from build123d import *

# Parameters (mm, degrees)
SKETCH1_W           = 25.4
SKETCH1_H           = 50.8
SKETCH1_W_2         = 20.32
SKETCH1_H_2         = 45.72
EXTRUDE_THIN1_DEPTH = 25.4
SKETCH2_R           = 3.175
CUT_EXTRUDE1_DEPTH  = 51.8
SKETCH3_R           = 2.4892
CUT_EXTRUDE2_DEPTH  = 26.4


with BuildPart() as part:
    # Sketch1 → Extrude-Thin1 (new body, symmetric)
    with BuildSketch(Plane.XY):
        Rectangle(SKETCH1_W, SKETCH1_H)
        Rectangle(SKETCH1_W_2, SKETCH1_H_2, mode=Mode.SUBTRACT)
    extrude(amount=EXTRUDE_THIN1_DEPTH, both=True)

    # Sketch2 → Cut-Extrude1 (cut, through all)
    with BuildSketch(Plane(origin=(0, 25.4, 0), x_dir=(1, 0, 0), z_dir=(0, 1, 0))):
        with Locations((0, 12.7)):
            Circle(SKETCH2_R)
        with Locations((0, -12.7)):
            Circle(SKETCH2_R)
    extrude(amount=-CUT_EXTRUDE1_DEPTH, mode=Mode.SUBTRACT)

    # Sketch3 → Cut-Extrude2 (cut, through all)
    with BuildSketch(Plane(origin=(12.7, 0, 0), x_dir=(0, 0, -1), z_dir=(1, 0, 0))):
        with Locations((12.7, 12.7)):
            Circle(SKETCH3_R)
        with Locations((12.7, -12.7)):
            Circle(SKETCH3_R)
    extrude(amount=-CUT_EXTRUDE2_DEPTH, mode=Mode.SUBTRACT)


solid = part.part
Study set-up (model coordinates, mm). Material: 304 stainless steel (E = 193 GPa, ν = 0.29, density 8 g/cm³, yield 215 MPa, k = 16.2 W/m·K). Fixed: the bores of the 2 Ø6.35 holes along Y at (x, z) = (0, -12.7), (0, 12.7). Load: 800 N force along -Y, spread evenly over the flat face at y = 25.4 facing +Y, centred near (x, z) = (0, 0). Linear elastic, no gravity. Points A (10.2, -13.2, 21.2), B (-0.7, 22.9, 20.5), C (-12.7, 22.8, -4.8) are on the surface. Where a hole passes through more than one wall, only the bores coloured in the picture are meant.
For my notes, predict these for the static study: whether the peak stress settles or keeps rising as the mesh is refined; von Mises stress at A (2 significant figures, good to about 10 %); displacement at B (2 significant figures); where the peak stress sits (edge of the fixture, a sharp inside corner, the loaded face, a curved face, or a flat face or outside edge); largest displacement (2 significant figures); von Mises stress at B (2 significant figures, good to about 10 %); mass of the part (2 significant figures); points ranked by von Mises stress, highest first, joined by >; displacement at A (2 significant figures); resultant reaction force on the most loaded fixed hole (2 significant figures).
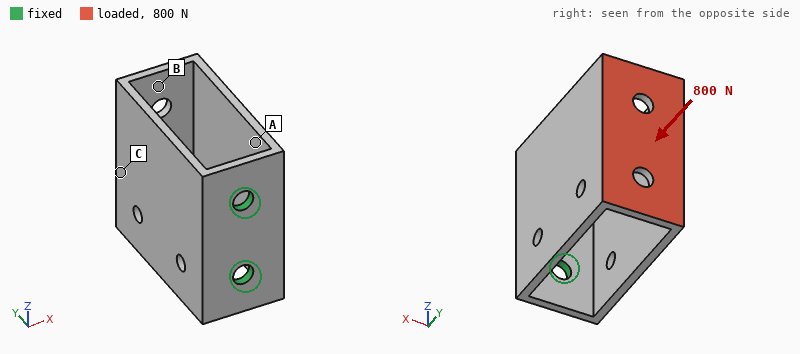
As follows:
keeps rising
13 MPa
15 µm
edge of the fixture
16 µm
33 MPa
140 g
B > A > C
11 µm
400 N
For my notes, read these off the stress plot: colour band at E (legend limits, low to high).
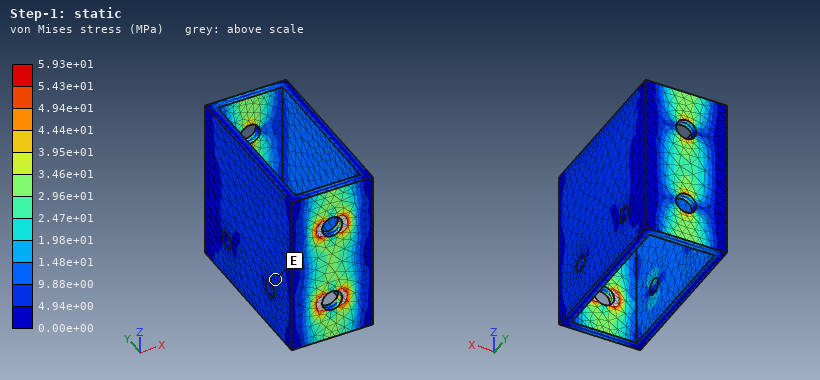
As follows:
4.94e+00 to 9.88e+00 MPa
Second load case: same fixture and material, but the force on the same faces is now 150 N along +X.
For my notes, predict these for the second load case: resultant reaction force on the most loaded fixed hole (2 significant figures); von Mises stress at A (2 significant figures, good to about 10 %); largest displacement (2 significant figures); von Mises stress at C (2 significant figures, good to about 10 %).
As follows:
75 N
15 MPa
0.13 mm
24 MPa
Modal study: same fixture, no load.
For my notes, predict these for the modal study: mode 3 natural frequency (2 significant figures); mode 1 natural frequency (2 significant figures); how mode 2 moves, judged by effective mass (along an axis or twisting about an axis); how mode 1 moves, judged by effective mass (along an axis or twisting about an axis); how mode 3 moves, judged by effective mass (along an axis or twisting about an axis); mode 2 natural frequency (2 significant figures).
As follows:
2400 Hz
710 Hz
along Z
along X
twisting about Y
2000 Hz
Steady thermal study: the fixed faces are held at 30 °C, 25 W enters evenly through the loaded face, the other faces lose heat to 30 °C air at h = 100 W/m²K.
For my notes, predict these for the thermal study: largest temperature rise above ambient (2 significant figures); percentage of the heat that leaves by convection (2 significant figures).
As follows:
75 K
98 %
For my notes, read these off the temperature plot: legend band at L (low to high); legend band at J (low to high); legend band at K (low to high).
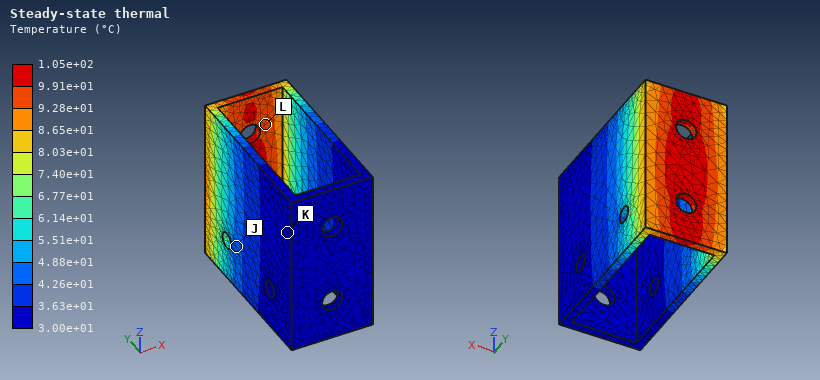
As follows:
9.28e+01 to 9.91e+01 °C
4.26e+01 to 4.88e+01 °C
3.00e+01 to 3.63e+01 °C
